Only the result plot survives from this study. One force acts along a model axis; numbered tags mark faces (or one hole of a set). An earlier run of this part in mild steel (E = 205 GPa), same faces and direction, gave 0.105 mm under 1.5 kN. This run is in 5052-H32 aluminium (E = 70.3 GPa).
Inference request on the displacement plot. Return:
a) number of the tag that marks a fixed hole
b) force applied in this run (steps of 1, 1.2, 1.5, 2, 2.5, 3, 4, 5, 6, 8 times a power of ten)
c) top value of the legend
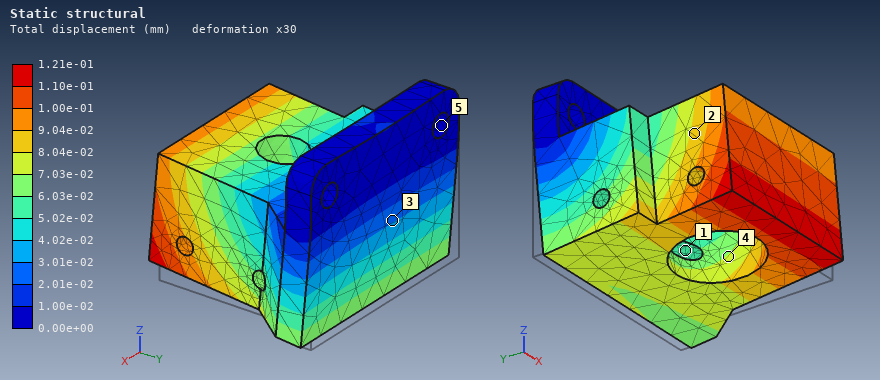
5
600 N
1.21e-01 mm
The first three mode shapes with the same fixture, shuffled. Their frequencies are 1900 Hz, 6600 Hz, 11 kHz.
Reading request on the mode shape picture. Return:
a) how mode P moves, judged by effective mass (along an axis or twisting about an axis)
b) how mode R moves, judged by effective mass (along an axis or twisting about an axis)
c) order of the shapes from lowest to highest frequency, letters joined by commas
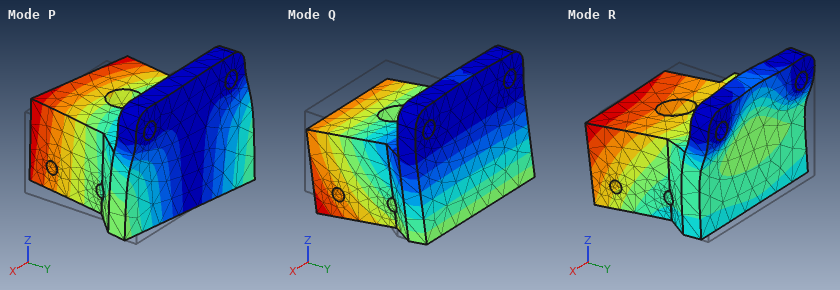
along X
along Y
Q, P, R
